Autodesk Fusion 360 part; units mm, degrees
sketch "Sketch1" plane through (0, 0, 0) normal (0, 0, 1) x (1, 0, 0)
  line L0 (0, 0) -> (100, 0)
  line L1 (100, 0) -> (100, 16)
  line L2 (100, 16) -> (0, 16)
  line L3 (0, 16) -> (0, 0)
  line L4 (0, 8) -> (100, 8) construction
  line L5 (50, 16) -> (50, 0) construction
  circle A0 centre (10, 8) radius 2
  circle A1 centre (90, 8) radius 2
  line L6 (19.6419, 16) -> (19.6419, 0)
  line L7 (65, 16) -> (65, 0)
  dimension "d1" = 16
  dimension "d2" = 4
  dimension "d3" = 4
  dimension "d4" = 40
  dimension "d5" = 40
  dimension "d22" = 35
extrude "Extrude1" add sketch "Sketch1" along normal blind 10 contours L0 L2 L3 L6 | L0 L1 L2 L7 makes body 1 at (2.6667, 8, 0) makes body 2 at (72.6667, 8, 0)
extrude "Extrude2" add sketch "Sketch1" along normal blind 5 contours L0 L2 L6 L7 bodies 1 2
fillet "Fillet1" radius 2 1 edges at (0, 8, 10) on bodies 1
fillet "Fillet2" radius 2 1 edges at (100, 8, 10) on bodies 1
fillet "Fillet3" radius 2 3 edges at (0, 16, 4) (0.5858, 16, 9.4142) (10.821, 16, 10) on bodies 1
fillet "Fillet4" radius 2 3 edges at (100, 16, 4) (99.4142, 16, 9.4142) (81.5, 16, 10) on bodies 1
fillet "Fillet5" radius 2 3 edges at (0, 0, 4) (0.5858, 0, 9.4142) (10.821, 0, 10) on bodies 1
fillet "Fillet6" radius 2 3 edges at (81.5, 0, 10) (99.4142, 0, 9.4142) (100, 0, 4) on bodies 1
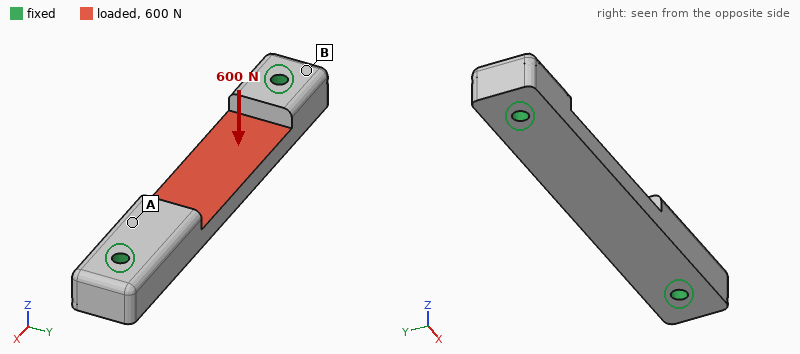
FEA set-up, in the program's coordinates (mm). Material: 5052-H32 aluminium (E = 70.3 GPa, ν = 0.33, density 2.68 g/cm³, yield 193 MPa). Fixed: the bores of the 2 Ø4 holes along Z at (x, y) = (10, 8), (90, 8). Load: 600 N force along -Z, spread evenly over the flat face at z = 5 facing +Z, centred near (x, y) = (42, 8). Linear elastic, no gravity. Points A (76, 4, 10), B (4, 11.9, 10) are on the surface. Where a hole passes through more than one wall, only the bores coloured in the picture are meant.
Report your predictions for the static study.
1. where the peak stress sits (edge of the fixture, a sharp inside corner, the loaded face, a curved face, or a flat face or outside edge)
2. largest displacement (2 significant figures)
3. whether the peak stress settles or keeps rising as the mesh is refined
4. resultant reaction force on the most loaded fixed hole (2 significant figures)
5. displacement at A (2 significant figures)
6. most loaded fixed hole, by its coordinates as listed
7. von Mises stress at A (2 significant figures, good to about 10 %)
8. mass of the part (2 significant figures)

edge of the fixture
38 µm
keeps rising
440 N
8.9 µm
(10, 8)
14 MPa
32 g
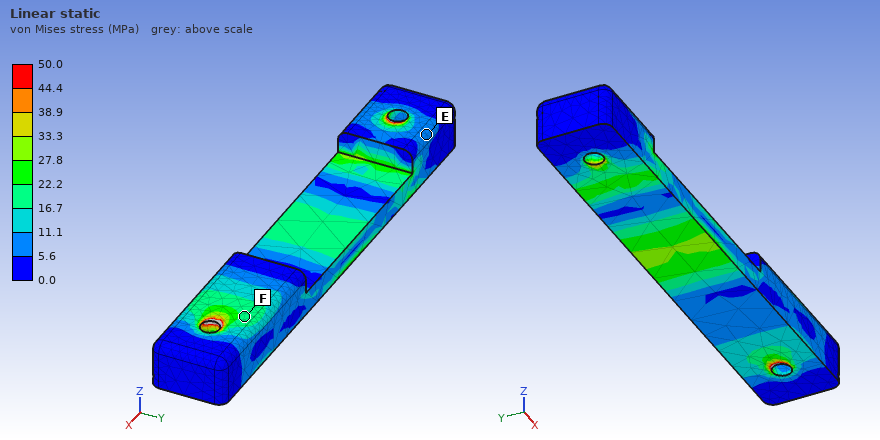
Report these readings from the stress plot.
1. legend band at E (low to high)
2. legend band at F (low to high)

5.6 to 11.1 MPa
16.7 to 22.2 MPa
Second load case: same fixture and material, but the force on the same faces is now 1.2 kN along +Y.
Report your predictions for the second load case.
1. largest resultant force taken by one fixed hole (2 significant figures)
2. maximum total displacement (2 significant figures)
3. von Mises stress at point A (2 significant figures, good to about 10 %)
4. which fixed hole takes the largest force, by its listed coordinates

730 N
37 µm
7.8 MPa
(10, 8)
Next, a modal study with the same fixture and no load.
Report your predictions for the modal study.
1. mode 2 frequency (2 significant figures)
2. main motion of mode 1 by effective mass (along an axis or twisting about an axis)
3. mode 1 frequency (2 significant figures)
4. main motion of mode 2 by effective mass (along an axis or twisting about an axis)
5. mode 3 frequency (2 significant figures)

9000 Hz
along Z
6700 Hz
along Y
14 kHz
